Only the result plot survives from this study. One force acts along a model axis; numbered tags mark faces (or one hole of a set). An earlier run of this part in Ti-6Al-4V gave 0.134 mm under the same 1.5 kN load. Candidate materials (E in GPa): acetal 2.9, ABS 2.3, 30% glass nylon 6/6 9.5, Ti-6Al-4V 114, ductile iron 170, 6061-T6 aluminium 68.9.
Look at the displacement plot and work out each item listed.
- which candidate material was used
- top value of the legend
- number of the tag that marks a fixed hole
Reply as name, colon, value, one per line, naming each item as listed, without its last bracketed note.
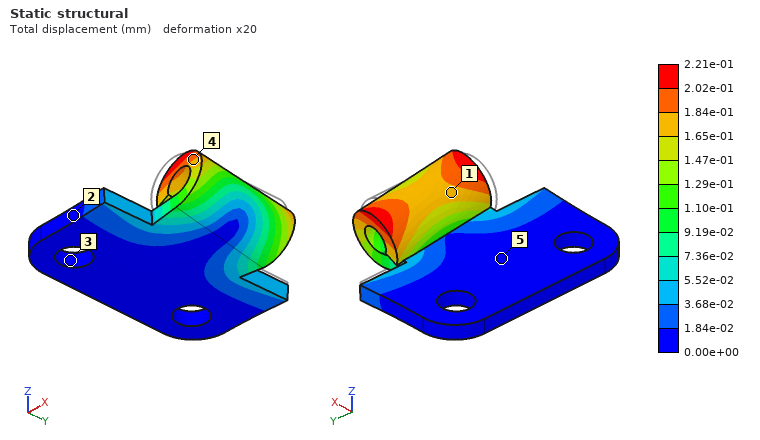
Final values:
which candidate material was used: 6061-T6 aluminium
top value of the legend: 2.21e-01 mm
number of the tag that marks a fixed hole: 3
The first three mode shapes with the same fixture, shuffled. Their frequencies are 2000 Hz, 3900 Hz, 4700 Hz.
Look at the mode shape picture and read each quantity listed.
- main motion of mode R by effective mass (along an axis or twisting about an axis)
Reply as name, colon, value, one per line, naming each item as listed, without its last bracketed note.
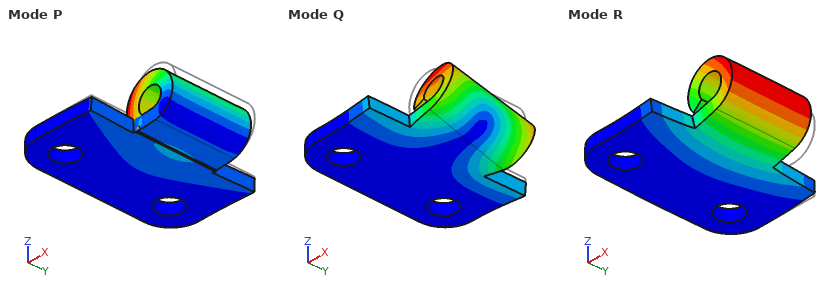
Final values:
main motion of mode R by effective mass: along Z
